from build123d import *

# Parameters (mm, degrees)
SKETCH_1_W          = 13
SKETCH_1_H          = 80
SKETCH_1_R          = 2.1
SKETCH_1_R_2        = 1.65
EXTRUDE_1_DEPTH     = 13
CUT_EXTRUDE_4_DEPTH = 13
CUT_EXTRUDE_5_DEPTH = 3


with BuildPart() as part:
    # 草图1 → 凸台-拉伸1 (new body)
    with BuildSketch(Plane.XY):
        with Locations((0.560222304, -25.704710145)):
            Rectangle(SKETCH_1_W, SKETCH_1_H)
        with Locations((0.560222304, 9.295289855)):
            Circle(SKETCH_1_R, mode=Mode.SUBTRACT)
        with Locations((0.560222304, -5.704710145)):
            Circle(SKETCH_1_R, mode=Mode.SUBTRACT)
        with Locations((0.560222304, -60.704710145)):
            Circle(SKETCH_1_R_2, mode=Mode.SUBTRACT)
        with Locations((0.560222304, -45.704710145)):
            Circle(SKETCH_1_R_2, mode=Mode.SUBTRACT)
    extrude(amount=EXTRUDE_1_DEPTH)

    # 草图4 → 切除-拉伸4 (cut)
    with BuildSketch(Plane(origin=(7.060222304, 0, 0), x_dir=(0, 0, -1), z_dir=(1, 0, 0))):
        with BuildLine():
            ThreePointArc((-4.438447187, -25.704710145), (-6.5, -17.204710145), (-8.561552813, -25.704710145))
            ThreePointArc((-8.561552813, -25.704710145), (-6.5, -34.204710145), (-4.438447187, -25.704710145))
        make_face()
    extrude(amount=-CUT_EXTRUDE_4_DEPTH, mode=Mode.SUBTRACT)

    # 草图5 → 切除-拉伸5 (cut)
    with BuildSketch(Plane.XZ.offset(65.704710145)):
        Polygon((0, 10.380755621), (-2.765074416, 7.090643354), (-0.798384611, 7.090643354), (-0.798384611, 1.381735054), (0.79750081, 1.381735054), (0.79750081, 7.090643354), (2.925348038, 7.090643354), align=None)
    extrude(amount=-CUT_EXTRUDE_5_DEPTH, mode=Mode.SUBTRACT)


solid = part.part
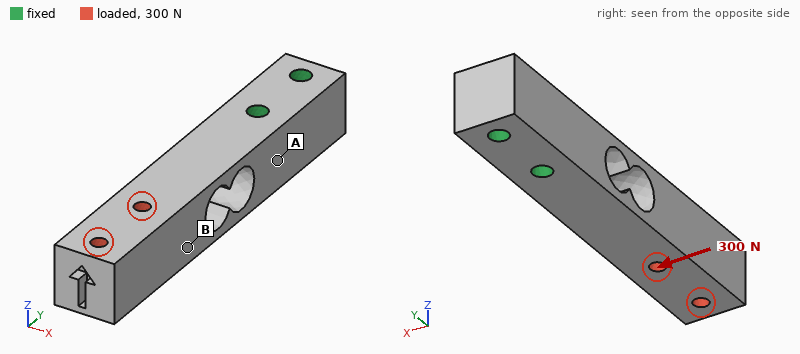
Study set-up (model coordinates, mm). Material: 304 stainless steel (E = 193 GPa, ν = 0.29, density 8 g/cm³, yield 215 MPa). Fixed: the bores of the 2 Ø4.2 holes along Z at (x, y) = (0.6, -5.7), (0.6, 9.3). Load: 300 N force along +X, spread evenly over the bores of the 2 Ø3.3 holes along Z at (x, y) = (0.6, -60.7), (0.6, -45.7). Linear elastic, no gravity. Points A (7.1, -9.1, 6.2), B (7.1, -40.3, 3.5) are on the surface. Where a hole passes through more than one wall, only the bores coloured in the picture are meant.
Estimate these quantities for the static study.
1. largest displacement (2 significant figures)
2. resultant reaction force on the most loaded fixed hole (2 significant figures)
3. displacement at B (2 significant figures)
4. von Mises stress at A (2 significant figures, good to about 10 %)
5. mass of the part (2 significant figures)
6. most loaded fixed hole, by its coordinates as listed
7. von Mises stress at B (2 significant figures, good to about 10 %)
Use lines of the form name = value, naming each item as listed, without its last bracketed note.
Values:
largest displacement = 70 µm
resultant reaction force on the most loaded fixed hole = 750 N
displacement at B = 32 µm
von Mises stress at A = 30 MPa
mass of the part = 90 g
most loaded fixed hole, by its coordinates as listed = (0.6, -5.7)
von Mises stress at B = 10 MPa
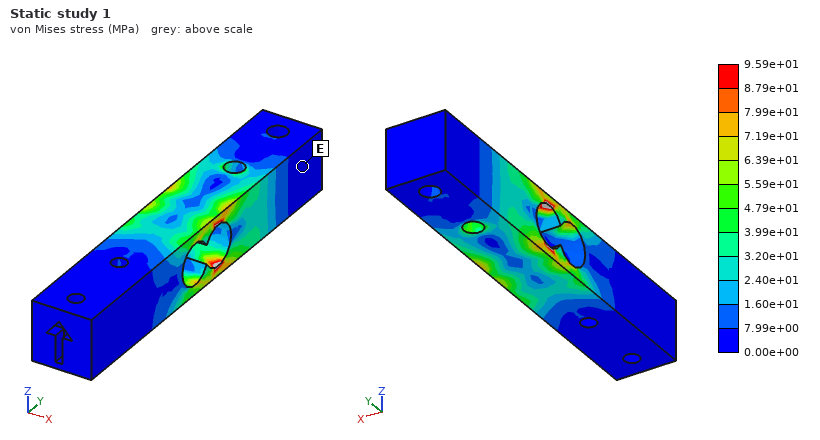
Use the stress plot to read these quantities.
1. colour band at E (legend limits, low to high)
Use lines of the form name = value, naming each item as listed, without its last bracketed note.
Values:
colour band at E = 0.00e+00 to 7.99e+00 MPa
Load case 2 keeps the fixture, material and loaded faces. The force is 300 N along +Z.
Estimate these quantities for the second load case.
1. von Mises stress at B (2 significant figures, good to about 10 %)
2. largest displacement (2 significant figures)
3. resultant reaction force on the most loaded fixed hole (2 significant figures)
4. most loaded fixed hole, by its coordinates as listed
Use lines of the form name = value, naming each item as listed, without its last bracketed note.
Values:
von Mises stress at B = 7.4 MPa
largest displacement = 60 µm
resultant reaction force on the most loaded fixed hole = 420 N
most loaded fixed hole, by its coordinates as listed = (0.6, -5.7)
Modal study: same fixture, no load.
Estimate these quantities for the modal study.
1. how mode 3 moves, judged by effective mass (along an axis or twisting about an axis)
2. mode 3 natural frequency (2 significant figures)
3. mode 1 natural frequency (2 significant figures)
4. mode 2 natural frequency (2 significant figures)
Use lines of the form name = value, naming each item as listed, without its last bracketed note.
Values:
how mode 3 moves, judged by effective mass = twisting about Y
mode 3 natural frequency = 7500 Hz
mode 1 natural frequency = 2000 Hz
mode 2 natural frequency = 2000 Hz
